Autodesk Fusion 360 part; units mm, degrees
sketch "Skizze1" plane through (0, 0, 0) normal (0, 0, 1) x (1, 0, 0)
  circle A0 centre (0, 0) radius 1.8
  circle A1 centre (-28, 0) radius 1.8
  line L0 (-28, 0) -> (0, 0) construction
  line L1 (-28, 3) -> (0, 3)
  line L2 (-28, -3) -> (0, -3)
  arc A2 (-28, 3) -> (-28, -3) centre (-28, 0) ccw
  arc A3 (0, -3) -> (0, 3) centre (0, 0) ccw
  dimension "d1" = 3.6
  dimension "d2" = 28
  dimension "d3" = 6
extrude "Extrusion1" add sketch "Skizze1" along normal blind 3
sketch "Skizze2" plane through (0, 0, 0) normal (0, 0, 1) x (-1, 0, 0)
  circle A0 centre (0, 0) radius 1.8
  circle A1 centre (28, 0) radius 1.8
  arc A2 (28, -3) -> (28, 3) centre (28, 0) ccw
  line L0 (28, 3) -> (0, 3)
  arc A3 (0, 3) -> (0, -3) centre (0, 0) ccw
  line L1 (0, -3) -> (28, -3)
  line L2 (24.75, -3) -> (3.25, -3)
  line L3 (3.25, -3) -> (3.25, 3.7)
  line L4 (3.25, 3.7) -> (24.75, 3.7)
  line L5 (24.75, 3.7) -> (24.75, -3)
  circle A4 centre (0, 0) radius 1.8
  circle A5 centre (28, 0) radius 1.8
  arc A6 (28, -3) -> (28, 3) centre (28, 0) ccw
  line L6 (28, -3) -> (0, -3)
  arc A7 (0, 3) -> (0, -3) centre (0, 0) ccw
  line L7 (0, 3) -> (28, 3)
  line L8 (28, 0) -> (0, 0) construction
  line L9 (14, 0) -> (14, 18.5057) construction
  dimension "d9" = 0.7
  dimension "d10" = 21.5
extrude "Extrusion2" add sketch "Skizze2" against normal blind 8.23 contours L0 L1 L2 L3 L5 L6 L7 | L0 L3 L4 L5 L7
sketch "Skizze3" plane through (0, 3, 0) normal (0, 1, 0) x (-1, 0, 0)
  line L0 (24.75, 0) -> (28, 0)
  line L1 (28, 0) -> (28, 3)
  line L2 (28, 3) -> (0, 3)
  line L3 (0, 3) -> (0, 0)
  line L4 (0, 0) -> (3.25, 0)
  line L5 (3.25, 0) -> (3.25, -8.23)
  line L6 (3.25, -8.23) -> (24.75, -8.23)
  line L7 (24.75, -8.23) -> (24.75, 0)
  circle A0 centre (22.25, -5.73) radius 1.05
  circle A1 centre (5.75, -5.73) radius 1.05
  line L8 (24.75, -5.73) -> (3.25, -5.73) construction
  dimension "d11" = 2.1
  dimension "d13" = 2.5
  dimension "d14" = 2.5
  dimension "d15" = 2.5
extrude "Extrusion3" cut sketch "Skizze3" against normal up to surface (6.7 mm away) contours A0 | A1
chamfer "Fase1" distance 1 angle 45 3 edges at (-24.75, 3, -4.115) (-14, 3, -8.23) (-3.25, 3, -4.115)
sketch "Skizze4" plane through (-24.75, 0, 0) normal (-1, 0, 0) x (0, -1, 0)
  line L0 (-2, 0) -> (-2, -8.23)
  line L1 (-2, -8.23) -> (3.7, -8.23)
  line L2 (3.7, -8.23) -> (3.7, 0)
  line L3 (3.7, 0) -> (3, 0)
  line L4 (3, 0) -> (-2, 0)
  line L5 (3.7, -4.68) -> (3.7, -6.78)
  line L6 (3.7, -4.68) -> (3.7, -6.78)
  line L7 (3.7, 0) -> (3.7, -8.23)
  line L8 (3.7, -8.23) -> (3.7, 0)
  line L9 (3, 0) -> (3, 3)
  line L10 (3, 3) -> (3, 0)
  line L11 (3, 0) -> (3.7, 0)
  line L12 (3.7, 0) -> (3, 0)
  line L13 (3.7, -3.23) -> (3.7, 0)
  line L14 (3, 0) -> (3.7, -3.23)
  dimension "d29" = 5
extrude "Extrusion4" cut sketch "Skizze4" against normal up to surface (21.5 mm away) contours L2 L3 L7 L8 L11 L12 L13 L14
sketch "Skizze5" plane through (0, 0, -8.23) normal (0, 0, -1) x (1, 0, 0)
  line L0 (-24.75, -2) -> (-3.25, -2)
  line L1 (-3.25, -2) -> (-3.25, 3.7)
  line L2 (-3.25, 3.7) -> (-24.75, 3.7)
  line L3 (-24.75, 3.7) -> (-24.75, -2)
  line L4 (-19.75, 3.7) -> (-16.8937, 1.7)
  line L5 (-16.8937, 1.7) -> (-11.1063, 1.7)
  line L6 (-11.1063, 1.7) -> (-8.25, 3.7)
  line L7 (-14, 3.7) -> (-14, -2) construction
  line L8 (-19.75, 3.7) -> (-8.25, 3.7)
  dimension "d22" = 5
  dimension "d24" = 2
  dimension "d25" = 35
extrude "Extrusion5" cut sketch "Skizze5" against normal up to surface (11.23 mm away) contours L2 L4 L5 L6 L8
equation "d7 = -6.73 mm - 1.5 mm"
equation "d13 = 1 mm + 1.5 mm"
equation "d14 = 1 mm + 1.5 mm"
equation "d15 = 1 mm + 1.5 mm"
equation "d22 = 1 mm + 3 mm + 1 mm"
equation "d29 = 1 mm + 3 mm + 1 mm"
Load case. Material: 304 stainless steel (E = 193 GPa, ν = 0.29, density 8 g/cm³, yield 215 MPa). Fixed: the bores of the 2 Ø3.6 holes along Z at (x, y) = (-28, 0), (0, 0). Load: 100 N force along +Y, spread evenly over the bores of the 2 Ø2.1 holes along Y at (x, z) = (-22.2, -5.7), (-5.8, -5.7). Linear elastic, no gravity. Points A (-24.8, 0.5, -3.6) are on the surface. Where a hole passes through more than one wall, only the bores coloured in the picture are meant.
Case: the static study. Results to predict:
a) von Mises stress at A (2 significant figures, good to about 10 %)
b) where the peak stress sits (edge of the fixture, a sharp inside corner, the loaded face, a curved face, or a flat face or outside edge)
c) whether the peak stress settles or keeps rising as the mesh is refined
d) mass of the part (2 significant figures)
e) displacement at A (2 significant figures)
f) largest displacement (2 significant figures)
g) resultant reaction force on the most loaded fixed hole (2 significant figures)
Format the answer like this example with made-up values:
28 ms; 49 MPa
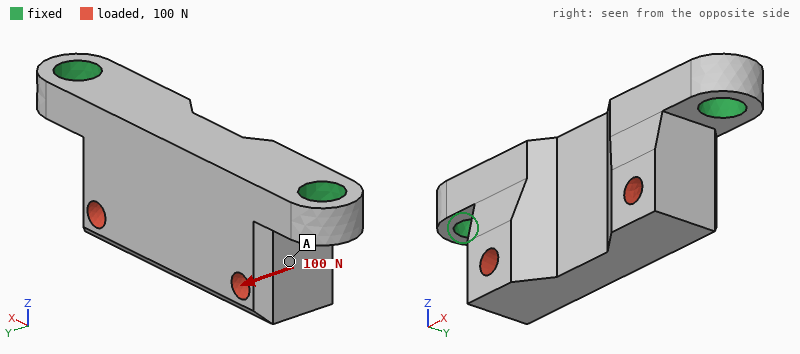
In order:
5.5 MPa; edge of the fixture; keeps rising; 12 g; 2.0 µm; 3.9 µm; 50 N
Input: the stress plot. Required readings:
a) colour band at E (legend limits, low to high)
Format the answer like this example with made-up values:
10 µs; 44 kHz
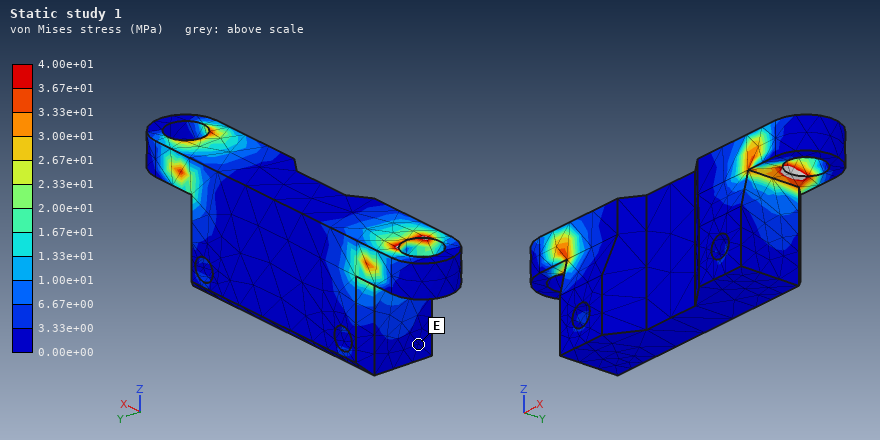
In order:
0.00e+00 to 3.33e+00 MPa
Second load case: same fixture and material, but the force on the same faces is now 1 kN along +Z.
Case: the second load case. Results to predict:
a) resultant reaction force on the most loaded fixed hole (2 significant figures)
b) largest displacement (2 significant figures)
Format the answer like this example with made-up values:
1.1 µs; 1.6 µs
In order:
540 N; 3.6 µm
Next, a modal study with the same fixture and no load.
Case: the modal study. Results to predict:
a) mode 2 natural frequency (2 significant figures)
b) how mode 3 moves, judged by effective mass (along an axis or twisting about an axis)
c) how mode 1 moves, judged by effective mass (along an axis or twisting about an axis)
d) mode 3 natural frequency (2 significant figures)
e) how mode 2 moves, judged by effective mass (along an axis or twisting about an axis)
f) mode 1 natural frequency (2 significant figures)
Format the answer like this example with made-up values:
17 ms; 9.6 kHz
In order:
29 kHz; along Y; along Y; 31 kHz; along Z; 12 kHz
